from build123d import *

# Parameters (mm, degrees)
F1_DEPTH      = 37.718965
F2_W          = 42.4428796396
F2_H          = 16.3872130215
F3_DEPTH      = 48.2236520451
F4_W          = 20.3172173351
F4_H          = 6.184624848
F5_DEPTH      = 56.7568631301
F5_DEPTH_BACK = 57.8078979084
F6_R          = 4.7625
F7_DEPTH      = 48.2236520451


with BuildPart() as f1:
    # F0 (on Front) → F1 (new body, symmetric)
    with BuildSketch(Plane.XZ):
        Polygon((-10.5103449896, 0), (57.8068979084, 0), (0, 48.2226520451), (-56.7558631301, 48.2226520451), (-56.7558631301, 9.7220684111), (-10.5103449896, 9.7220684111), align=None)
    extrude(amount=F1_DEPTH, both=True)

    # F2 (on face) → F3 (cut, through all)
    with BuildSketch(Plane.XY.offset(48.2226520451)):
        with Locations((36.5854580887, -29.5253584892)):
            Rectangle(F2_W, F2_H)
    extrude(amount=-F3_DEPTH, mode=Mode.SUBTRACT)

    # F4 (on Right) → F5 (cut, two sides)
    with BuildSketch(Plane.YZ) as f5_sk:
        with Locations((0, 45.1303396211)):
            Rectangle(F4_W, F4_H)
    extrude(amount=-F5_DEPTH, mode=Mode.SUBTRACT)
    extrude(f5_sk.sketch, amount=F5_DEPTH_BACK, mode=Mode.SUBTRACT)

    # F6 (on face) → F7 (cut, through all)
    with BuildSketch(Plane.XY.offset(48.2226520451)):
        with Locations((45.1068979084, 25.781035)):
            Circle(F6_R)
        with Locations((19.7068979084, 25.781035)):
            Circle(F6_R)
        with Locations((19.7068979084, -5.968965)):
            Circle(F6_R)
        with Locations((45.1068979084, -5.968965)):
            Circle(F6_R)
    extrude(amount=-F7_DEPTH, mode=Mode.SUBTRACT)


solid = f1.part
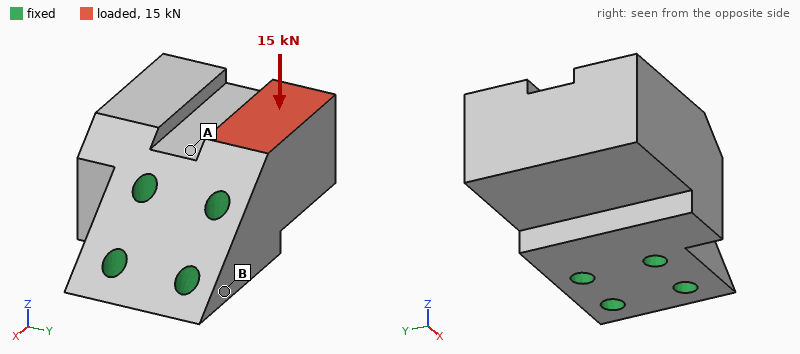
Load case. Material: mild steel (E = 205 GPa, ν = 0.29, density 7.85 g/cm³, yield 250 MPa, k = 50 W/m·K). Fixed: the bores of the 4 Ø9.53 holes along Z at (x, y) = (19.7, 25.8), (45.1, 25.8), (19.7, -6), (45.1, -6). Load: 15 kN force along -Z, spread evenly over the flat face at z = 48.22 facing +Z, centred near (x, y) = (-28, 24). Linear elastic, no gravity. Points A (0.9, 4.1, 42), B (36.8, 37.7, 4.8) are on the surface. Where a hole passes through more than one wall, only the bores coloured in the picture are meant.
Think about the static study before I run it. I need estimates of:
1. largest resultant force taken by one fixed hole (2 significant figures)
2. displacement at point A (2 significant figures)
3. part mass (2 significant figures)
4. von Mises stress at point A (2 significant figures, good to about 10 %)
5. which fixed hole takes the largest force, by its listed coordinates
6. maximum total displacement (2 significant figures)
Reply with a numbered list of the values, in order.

1. 12 kN
2. 8.4 µm
3. 2.0 kg
4. 24 MPa
5. (19.7, 25.8)
6. 38 µm
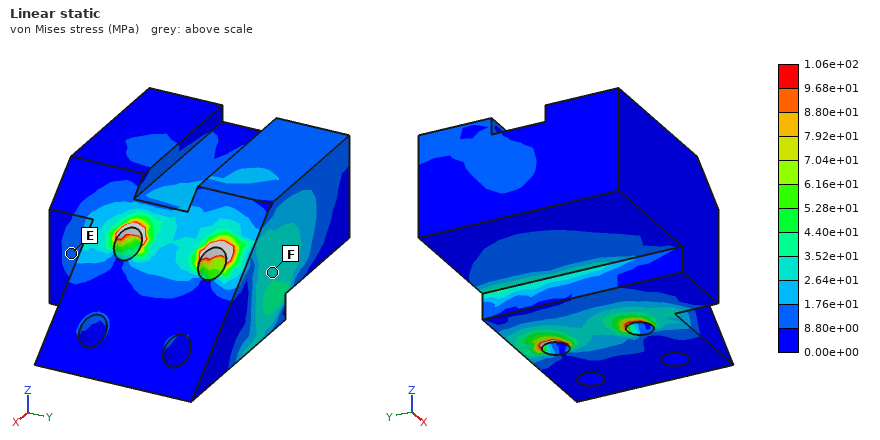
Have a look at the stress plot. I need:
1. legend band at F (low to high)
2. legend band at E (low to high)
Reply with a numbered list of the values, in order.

1. 2.64e+01 to 3.52e+01 MPa
2. 8.80e+00 to 1.76e+01 MPa
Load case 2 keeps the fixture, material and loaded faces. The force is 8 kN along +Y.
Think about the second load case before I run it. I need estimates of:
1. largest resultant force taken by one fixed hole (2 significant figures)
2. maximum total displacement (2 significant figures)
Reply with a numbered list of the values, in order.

1. 11 kN
2. 13 µm
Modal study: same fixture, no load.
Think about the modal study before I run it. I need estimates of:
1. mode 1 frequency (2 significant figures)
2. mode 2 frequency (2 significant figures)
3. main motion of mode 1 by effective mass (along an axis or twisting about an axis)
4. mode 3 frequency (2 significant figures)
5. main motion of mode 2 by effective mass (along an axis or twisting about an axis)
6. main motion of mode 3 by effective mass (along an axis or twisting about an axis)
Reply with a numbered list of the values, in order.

1. 3800 Hz
2. 4900 Hz
3. along Z
4. 7100 Hz
5. along Y
6. twisting about X
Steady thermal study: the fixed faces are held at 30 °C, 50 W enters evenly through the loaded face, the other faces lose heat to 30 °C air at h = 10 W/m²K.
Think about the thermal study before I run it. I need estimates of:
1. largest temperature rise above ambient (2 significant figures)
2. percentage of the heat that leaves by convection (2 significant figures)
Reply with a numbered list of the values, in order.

1. 32 K
2. 5.1 %
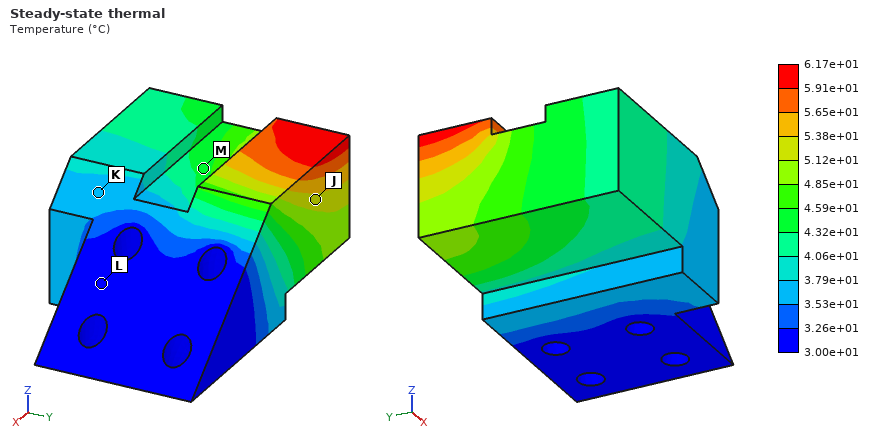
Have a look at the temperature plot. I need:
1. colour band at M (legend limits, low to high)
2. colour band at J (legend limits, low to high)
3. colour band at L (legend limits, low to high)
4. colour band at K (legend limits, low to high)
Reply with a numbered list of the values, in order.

1. 4.32e+01 to 4.59e+01 °C
2. 5.12e+01 to 5.38e+01 °C
3. 3.00e+01 to 3.26e+01 °C
4. 3.53e+01 to 3.79e+01 °C
